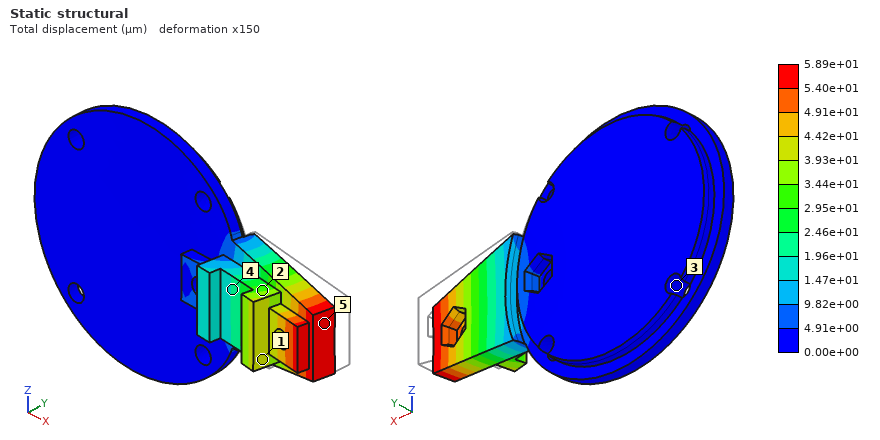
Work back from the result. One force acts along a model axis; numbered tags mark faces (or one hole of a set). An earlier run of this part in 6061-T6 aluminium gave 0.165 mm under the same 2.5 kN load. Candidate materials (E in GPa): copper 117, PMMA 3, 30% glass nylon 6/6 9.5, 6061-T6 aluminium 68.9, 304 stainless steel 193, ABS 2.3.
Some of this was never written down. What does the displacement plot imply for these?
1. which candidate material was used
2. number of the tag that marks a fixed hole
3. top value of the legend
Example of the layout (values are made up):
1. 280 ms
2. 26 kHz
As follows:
1. 304 stainless steel
2. 3
3. 5.89e+01 µm
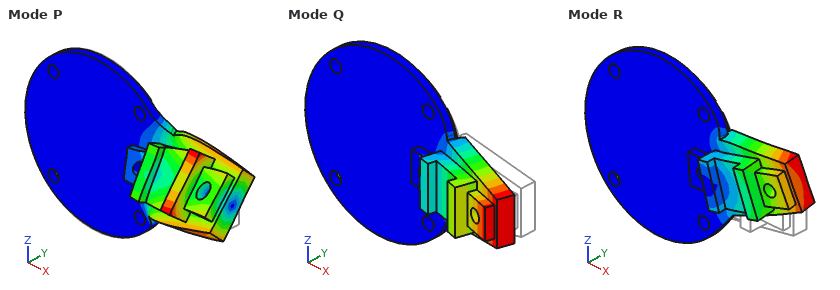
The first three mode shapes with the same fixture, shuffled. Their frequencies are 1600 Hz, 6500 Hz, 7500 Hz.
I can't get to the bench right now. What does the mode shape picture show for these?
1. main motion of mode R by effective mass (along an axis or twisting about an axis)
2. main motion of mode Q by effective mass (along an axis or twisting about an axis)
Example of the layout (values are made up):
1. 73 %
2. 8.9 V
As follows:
1. along Z
2. along Y
